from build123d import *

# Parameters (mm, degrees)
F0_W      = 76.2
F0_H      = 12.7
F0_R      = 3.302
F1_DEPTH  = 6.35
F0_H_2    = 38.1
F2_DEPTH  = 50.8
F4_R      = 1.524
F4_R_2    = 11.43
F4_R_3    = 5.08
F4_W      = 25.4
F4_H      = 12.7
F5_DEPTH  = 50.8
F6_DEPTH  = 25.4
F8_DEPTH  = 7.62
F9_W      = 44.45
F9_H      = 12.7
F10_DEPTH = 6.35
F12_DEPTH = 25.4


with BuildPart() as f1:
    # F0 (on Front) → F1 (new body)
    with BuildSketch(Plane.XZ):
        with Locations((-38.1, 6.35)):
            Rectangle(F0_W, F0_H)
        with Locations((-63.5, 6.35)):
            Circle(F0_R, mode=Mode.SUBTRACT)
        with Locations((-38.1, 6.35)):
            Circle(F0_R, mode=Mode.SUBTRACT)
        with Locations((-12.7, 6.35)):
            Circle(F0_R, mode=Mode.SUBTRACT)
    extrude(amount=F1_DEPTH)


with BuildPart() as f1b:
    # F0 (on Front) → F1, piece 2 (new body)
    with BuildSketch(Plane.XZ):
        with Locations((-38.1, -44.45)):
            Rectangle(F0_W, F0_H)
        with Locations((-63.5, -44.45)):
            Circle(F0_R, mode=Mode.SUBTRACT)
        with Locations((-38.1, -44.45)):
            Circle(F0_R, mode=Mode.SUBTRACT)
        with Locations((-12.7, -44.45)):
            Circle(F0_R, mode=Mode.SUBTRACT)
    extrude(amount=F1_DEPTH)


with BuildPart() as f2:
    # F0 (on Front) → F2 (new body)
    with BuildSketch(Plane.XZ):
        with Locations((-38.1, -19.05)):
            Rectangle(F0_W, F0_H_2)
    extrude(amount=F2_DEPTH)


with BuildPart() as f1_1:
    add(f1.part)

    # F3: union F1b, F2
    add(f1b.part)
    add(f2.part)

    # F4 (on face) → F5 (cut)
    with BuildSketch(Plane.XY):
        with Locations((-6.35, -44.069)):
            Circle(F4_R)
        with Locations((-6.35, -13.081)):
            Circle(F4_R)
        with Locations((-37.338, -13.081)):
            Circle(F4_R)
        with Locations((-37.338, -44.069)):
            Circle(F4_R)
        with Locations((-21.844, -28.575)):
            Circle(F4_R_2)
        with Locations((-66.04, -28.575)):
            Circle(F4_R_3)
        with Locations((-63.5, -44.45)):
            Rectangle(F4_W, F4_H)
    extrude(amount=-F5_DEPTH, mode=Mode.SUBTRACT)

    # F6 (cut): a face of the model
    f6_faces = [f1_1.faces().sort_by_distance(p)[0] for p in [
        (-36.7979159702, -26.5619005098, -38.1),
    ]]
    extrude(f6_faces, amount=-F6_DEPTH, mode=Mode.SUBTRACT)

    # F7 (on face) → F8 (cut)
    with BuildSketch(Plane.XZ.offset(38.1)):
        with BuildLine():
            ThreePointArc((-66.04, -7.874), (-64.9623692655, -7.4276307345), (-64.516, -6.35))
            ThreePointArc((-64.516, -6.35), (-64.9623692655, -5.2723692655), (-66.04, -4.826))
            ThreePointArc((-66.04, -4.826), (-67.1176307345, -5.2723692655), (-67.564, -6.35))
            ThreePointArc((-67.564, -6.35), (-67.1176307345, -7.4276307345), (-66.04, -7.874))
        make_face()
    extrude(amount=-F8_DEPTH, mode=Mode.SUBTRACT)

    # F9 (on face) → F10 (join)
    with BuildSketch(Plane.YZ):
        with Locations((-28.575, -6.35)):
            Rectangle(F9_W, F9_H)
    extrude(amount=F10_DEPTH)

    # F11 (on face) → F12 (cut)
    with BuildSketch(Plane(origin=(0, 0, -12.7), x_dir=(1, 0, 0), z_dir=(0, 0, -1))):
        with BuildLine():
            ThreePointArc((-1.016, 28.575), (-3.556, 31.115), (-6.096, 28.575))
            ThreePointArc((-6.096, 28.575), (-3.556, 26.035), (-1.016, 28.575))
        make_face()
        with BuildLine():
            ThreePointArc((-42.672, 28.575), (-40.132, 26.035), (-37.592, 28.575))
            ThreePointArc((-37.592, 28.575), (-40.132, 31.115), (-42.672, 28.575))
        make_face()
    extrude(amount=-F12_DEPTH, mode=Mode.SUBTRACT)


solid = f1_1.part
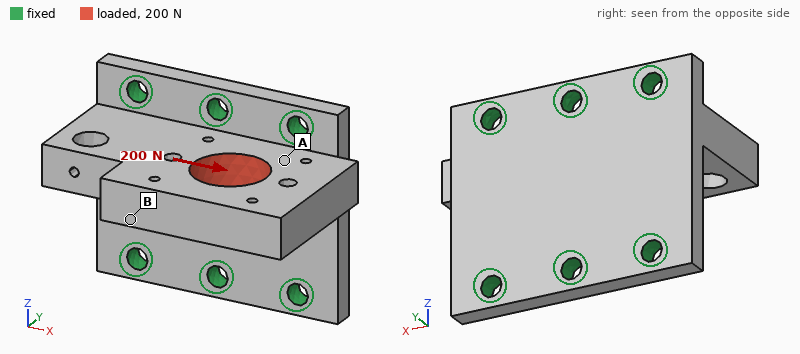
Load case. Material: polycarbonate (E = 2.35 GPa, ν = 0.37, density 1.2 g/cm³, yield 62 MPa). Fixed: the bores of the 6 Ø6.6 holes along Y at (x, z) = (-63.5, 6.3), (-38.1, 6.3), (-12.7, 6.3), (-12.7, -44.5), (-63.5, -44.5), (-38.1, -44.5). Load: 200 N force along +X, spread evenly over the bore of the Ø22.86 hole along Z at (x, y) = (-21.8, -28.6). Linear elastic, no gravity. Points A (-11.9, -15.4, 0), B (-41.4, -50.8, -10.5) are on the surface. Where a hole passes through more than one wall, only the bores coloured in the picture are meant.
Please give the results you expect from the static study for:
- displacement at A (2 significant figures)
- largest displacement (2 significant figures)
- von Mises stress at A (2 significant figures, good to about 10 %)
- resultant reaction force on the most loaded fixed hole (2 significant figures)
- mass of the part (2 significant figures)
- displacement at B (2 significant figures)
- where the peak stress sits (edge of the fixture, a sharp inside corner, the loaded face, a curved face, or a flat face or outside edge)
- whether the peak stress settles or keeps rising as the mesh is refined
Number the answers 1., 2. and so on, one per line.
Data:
1. 20 µm
2. 61 µm
3. 0.58 MPa
4. 99 N
5. 78 g
6. 44 µm
7. edge of the fixture
8. keeps rising
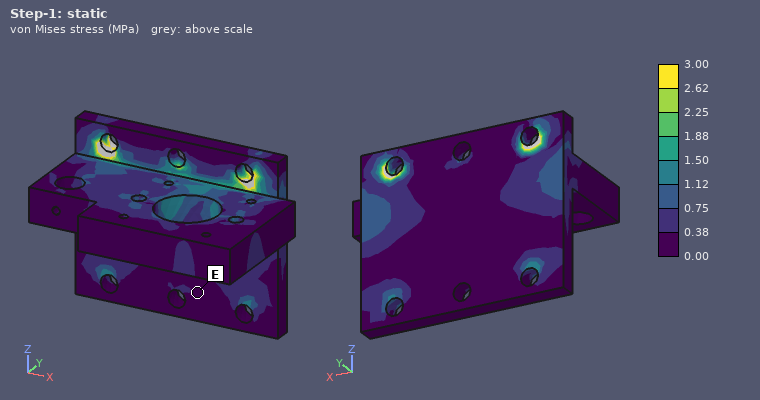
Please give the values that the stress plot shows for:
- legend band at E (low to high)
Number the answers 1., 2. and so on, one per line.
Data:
1. 0.00 to 0.38 MPa
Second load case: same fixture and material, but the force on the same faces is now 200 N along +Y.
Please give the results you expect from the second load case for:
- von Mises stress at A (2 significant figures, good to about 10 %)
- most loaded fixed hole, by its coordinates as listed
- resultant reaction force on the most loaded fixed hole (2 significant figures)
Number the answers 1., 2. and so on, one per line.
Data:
1. 0.80 MPa
2. (-12.7, 6.3)
3. 110 N
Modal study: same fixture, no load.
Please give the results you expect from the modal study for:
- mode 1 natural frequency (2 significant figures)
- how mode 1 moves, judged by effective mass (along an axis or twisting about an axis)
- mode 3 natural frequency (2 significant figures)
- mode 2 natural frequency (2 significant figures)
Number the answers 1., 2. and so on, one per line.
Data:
1. 830 Hz
2. along Z
3. 1900 Hz
4. 1500 Hz
